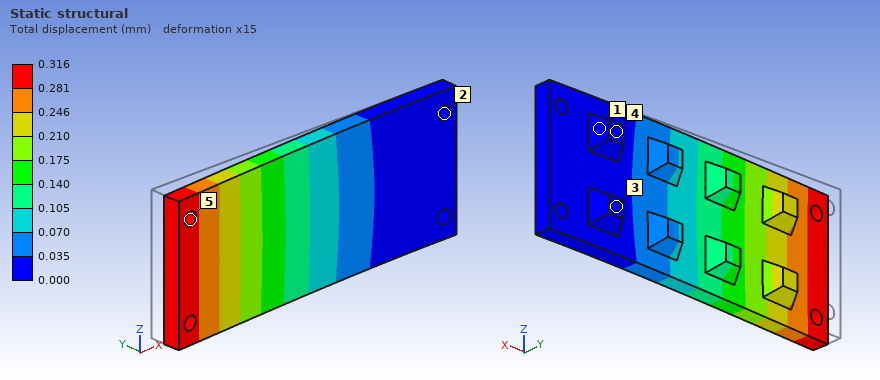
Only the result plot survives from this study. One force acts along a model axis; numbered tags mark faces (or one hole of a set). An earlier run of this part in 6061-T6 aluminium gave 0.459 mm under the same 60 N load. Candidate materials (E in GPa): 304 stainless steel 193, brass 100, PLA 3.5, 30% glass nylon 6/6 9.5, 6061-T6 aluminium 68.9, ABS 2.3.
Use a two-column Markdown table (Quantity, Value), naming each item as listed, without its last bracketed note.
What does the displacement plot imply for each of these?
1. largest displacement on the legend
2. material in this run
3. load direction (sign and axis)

| Quantity | Value |
|---|---|
| largest displacement on the legend | 0.316 mm |
| material in this run | brass |
| load direction | -Y |
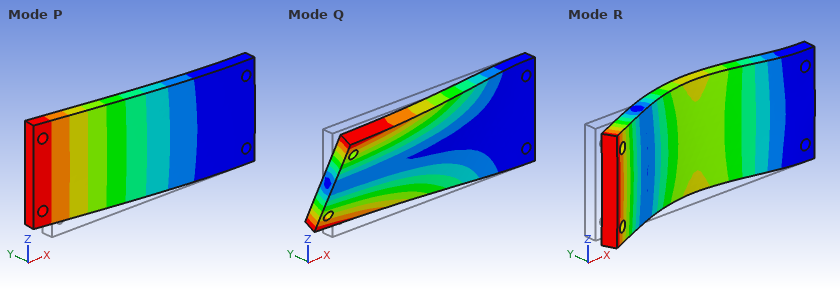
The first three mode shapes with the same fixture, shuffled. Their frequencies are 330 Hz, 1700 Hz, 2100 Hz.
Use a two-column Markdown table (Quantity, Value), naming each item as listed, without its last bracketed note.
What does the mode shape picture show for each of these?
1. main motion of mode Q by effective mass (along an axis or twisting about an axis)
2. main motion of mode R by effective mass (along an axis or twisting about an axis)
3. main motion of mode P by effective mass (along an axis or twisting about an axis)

| Quantity | Value |
|---|---|
| main motion of mode Q by effective mass | twisting about X |
| main motion of mode R by effective mass | along Y |
| main motion of mode P by effective mass | along Y |
